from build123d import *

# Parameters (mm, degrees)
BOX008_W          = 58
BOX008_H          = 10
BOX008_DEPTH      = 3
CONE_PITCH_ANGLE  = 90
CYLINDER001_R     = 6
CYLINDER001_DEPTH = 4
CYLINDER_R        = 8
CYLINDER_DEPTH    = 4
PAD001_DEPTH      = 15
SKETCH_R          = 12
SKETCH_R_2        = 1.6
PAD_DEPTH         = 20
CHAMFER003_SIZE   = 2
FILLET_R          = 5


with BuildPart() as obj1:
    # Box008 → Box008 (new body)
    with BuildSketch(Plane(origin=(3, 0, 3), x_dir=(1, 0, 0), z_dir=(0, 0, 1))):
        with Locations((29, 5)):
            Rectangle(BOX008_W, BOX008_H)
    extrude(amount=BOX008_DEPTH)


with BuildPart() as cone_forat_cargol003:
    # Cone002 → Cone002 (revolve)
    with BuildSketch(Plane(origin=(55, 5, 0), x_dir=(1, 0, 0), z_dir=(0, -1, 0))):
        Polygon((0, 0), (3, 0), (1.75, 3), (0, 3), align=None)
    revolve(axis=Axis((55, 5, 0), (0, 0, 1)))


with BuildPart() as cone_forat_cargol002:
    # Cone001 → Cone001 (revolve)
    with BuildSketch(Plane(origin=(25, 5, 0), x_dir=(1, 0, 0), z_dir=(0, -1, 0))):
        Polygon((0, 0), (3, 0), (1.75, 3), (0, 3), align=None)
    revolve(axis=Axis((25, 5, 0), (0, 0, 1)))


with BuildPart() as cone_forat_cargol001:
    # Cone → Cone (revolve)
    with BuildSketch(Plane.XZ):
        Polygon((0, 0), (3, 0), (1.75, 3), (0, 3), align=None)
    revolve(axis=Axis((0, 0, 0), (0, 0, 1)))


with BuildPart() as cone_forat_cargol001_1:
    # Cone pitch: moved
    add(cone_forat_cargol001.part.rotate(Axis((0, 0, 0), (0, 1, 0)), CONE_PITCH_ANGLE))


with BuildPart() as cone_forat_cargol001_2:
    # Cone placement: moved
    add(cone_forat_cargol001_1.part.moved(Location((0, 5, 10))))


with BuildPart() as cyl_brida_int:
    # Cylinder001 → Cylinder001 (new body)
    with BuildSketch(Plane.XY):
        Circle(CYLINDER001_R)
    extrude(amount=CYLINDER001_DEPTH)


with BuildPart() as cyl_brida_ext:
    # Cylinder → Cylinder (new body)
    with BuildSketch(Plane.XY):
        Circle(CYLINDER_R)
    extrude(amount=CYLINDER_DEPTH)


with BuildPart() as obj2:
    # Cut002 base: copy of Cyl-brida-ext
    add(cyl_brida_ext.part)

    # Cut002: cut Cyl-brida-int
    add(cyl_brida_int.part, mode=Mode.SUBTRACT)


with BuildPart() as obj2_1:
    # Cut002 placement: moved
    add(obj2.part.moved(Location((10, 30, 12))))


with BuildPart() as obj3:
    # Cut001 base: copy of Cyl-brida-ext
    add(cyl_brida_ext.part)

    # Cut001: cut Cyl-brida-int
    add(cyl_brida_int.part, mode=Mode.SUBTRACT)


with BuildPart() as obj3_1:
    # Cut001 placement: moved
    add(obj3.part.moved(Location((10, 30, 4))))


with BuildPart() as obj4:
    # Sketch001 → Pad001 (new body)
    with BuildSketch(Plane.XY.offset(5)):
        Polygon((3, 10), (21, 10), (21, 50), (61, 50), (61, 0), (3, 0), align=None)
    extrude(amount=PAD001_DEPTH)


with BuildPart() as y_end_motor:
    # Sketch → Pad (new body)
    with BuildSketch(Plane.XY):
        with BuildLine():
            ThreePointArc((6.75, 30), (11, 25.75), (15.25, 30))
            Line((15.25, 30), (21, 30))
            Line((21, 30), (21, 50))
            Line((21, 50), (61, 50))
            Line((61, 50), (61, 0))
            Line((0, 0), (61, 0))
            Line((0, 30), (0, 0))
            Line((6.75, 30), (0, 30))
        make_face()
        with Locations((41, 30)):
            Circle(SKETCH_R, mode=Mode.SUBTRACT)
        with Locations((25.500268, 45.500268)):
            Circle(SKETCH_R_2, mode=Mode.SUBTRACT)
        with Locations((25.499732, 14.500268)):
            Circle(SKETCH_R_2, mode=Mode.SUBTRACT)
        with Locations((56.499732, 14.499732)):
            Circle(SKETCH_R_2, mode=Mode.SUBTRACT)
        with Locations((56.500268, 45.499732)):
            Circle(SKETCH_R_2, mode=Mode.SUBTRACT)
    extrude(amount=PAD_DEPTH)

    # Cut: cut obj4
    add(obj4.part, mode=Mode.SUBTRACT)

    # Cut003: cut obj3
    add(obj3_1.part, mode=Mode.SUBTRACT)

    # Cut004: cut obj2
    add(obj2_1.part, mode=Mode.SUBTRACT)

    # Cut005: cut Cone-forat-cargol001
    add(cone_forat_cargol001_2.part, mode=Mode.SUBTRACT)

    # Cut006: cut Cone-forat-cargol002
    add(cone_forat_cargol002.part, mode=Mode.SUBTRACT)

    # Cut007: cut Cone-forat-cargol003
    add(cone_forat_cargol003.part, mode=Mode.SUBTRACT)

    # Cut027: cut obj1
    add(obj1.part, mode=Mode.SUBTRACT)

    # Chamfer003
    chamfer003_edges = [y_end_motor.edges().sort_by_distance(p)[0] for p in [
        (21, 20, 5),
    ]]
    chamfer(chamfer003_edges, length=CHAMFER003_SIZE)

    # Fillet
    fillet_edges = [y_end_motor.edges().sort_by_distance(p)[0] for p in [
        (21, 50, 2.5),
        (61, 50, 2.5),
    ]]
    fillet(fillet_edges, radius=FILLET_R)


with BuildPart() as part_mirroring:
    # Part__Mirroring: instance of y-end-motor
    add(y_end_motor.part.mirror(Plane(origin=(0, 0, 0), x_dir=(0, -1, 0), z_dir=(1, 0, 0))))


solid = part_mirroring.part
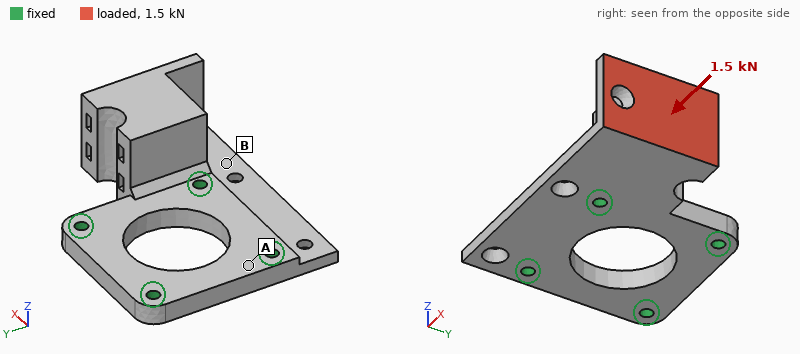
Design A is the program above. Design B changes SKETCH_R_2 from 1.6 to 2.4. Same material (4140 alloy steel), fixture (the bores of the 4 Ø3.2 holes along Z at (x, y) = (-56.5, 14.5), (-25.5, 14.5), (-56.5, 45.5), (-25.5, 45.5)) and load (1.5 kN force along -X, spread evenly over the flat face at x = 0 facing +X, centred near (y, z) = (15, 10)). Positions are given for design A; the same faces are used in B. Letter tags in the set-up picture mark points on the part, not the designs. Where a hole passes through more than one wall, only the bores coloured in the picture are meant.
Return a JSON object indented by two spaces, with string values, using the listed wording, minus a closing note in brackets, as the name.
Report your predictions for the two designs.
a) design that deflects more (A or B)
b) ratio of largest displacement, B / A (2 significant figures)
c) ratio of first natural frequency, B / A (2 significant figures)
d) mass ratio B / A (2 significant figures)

{
  "design that deflects more": "A",
  "ratio of largest displacement, B / A": "0.83",
  "ratio of first natural frequency, B / A": "1.1",
  "mass ratio B / A": "0.99"
}
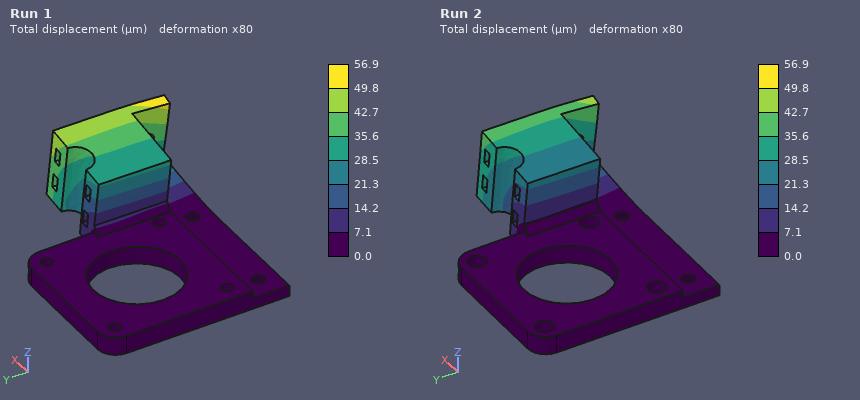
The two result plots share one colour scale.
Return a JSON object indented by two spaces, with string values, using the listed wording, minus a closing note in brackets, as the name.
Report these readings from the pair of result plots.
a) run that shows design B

{
  "run that shows design B": "Run 2"
}
